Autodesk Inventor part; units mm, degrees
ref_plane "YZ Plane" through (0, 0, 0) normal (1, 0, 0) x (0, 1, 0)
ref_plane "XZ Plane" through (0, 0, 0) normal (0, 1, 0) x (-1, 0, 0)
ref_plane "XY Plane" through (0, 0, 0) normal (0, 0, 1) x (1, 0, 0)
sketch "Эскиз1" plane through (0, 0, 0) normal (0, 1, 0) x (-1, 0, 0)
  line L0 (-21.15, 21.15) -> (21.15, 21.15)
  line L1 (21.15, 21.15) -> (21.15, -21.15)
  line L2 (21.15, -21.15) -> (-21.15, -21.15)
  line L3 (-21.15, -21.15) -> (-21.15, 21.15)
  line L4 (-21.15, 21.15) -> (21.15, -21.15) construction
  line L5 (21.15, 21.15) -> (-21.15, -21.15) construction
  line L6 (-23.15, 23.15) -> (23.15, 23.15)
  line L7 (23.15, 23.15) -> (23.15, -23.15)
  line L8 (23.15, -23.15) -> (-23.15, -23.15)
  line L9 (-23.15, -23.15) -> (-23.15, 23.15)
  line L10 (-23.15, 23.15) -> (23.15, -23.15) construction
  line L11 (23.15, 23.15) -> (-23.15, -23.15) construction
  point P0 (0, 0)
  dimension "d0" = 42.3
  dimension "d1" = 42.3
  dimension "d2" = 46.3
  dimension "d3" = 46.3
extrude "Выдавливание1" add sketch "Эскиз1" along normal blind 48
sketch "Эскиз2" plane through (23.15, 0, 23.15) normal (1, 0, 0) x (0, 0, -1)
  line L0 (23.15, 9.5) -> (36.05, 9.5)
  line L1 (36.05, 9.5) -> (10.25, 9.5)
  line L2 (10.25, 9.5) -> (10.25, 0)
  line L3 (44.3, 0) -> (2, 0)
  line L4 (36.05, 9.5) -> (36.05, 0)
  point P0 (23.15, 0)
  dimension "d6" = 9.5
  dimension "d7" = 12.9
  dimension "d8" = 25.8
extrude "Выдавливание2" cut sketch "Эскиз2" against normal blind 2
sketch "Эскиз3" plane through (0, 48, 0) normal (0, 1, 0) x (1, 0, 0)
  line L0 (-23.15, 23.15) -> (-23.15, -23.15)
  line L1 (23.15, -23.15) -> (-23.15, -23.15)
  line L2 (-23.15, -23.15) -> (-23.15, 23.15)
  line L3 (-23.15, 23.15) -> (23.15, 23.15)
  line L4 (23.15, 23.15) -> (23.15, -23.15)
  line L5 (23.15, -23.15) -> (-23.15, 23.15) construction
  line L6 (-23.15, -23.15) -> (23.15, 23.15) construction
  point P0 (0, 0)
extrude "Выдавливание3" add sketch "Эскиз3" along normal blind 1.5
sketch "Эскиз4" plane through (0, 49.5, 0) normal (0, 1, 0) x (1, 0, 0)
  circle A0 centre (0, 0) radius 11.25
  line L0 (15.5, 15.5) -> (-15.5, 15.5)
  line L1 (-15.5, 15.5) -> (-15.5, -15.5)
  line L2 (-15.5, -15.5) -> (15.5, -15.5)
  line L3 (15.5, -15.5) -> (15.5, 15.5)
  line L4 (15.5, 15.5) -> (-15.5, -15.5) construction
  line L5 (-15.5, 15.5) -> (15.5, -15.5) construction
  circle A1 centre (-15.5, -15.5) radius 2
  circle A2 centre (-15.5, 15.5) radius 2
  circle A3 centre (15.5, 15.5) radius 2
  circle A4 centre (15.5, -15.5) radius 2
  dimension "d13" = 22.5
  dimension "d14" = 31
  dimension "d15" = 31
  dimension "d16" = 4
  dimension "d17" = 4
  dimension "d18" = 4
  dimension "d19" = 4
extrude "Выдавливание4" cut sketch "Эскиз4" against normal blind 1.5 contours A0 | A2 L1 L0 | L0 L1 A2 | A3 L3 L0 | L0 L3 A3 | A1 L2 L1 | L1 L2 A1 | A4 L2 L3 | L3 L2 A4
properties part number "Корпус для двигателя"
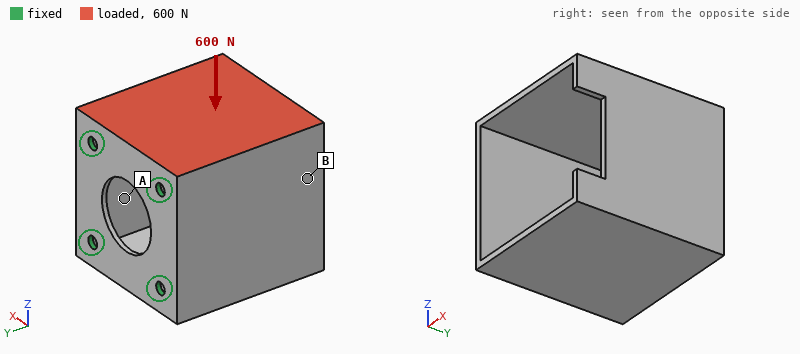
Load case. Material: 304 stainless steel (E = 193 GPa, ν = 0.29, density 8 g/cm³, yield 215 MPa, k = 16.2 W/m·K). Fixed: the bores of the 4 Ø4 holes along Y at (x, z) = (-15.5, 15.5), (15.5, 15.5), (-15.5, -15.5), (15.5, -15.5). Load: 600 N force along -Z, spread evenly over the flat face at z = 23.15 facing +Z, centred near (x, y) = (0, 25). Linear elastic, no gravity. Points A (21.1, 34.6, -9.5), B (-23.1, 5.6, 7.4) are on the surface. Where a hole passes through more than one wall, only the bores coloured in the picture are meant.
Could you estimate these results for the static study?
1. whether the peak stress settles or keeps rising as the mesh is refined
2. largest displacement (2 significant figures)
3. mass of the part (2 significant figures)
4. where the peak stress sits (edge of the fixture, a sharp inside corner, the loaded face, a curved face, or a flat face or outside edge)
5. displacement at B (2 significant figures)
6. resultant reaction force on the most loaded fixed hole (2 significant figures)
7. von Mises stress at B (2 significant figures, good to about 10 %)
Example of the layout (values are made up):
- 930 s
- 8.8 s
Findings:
- keeps rising
- 64 µm
- 150 g
- edge of the fixture
- 21 µm
- 300 N
- 17 MPa
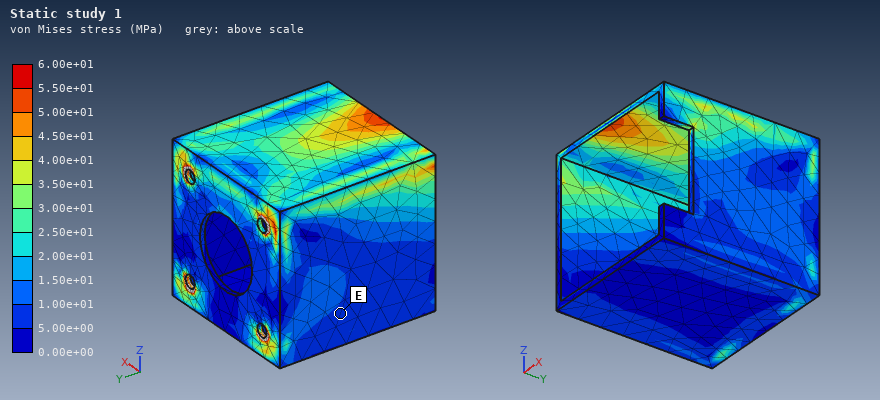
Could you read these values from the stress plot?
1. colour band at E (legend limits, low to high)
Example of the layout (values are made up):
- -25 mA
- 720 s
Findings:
- 5.00e+00 to 1.00e+01 MPa
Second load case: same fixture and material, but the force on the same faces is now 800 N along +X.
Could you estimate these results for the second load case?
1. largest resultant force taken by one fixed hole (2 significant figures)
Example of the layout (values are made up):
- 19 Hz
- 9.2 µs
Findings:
- 670 N
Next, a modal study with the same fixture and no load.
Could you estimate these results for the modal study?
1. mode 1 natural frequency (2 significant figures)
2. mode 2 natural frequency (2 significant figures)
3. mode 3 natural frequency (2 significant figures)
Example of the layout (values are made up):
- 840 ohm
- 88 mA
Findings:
- 2700 Hz
- 2800 Hz
- 2900 Hz
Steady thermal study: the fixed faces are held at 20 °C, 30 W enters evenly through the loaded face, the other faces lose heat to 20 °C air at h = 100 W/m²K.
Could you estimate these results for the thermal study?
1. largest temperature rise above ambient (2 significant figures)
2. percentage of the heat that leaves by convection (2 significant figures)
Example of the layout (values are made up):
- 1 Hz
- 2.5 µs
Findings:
- 82 K
- 86 %
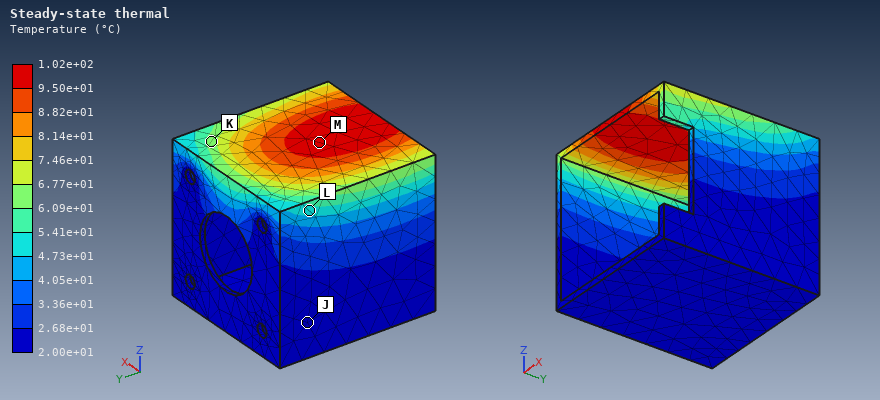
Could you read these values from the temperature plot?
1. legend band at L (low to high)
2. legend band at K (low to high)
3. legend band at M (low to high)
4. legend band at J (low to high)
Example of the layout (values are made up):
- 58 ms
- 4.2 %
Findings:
- 4.73e+01 to 5.41e+01 °C
- 6.09e+01 to 6.77e+01 °C
- 9.50e+01 to 1.02e+02 °C
- 2.00e+01 to 2.68e+01 °C
